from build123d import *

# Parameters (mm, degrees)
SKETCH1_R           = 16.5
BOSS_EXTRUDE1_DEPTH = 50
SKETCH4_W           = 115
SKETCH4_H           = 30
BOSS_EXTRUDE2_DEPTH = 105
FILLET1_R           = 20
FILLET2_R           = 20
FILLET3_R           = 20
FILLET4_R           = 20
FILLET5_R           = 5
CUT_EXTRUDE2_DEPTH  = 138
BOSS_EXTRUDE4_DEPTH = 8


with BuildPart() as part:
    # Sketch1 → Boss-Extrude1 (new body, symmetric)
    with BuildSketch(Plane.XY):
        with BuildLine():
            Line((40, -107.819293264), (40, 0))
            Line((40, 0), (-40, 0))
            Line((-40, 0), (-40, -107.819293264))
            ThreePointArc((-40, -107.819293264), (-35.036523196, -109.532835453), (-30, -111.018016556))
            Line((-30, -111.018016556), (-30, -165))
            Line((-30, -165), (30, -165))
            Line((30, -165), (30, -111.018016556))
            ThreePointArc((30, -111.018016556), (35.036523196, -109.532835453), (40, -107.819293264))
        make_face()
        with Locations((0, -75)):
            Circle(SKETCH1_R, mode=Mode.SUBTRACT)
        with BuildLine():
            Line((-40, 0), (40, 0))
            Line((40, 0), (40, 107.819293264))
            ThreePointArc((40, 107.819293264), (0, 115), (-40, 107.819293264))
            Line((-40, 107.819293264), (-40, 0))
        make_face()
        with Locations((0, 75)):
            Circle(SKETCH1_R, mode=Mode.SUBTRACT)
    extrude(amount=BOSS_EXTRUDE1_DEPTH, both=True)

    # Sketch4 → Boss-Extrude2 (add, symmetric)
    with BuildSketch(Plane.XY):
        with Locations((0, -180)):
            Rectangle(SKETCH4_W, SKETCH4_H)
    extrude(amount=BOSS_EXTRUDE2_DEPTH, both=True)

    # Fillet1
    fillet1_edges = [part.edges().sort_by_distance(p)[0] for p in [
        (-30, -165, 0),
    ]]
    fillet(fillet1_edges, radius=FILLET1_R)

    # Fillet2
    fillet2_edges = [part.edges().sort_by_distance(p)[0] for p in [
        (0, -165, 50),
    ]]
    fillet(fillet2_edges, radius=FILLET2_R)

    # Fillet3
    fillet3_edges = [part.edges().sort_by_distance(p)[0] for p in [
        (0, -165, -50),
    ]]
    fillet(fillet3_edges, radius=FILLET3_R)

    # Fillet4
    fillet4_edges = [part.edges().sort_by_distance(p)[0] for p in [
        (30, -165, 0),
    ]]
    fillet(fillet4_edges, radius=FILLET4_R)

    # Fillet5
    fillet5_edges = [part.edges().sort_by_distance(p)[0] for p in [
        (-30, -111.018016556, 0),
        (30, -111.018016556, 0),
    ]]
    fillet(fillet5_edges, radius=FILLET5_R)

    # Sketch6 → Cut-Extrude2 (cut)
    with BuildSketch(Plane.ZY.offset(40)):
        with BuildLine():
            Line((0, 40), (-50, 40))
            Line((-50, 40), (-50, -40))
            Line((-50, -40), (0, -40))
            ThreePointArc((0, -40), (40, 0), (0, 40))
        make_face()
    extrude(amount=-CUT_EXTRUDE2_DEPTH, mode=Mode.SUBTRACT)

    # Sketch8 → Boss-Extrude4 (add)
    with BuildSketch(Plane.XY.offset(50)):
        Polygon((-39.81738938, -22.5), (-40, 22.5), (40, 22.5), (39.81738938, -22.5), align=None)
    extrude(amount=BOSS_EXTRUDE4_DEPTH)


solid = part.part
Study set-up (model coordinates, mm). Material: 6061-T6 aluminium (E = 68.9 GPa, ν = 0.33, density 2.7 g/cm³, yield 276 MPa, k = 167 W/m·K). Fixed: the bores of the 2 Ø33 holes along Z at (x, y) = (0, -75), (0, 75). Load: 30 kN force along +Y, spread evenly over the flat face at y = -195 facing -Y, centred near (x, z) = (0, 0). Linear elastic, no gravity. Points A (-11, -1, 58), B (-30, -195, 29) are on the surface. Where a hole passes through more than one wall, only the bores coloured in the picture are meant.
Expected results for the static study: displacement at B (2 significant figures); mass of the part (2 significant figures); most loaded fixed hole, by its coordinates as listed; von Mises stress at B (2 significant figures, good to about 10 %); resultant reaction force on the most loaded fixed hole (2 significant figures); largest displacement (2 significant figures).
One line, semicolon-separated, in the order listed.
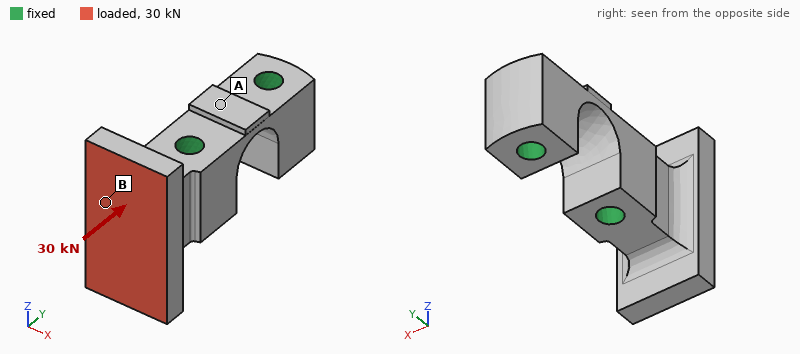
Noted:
6.6 µm; 5.9 kg; (0, -75); 7.5 MPa; 30 kN; 30 µm
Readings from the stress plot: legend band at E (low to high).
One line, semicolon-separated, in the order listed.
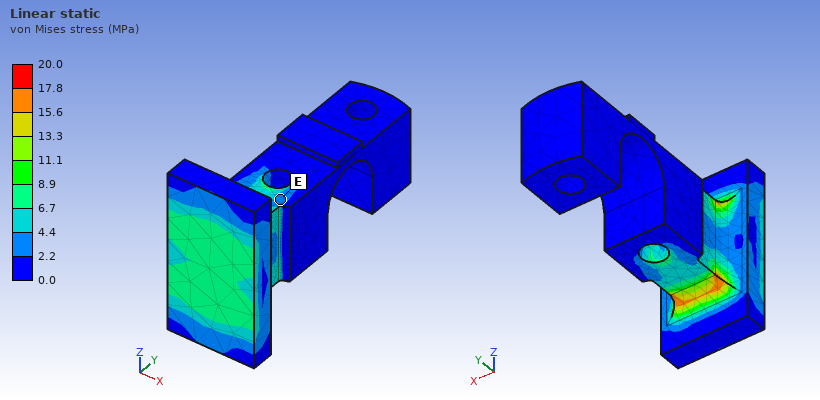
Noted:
2.2 to 4.4 MPa
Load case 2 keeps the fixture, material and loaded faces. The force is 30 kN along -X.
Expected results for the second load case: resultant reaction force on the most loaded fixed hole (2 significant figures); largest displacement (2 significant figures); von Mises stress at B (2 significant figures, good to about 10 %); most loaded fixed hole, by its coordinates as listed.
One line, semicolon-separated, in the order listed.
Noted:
32 kN; 0.16 mm; 5.8 MPa; (0, -75)
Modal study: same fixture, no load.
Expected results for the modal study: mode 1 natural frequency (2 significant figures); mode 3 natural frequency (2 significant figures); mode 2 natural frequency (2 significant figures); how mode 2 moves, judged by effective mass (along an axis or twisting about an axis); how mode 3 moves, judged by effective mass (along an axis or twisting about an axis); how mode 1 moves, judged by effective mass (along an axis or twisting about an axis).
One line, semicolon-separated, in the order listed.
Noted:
1800 Hz; 2300 Hz; 2100 Hz; twisting about Y; along Z; along X
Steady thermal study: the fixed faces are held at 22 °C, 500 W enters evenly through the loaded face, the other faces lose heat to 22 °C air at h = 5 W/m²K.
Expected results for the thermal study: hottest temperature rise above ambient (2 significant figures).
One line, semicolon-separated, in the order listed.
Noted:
49 K
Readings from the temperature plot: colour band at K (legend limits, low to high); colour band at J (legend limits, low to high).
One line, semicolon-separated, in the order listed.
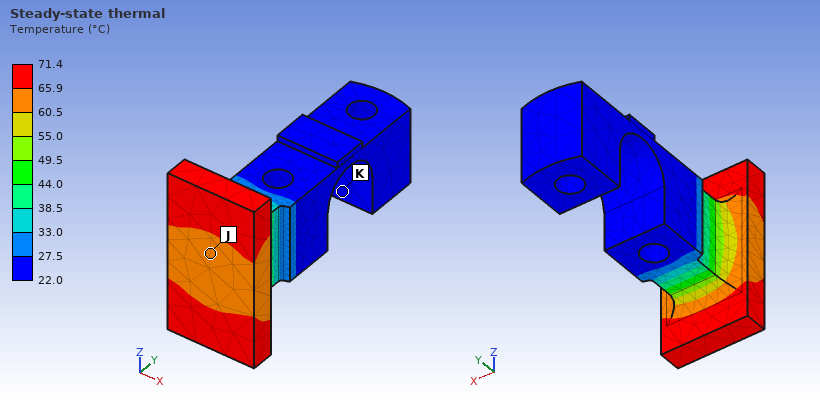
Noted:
22.0 to 27.5 °C; 60.5 to 65.9 °C
